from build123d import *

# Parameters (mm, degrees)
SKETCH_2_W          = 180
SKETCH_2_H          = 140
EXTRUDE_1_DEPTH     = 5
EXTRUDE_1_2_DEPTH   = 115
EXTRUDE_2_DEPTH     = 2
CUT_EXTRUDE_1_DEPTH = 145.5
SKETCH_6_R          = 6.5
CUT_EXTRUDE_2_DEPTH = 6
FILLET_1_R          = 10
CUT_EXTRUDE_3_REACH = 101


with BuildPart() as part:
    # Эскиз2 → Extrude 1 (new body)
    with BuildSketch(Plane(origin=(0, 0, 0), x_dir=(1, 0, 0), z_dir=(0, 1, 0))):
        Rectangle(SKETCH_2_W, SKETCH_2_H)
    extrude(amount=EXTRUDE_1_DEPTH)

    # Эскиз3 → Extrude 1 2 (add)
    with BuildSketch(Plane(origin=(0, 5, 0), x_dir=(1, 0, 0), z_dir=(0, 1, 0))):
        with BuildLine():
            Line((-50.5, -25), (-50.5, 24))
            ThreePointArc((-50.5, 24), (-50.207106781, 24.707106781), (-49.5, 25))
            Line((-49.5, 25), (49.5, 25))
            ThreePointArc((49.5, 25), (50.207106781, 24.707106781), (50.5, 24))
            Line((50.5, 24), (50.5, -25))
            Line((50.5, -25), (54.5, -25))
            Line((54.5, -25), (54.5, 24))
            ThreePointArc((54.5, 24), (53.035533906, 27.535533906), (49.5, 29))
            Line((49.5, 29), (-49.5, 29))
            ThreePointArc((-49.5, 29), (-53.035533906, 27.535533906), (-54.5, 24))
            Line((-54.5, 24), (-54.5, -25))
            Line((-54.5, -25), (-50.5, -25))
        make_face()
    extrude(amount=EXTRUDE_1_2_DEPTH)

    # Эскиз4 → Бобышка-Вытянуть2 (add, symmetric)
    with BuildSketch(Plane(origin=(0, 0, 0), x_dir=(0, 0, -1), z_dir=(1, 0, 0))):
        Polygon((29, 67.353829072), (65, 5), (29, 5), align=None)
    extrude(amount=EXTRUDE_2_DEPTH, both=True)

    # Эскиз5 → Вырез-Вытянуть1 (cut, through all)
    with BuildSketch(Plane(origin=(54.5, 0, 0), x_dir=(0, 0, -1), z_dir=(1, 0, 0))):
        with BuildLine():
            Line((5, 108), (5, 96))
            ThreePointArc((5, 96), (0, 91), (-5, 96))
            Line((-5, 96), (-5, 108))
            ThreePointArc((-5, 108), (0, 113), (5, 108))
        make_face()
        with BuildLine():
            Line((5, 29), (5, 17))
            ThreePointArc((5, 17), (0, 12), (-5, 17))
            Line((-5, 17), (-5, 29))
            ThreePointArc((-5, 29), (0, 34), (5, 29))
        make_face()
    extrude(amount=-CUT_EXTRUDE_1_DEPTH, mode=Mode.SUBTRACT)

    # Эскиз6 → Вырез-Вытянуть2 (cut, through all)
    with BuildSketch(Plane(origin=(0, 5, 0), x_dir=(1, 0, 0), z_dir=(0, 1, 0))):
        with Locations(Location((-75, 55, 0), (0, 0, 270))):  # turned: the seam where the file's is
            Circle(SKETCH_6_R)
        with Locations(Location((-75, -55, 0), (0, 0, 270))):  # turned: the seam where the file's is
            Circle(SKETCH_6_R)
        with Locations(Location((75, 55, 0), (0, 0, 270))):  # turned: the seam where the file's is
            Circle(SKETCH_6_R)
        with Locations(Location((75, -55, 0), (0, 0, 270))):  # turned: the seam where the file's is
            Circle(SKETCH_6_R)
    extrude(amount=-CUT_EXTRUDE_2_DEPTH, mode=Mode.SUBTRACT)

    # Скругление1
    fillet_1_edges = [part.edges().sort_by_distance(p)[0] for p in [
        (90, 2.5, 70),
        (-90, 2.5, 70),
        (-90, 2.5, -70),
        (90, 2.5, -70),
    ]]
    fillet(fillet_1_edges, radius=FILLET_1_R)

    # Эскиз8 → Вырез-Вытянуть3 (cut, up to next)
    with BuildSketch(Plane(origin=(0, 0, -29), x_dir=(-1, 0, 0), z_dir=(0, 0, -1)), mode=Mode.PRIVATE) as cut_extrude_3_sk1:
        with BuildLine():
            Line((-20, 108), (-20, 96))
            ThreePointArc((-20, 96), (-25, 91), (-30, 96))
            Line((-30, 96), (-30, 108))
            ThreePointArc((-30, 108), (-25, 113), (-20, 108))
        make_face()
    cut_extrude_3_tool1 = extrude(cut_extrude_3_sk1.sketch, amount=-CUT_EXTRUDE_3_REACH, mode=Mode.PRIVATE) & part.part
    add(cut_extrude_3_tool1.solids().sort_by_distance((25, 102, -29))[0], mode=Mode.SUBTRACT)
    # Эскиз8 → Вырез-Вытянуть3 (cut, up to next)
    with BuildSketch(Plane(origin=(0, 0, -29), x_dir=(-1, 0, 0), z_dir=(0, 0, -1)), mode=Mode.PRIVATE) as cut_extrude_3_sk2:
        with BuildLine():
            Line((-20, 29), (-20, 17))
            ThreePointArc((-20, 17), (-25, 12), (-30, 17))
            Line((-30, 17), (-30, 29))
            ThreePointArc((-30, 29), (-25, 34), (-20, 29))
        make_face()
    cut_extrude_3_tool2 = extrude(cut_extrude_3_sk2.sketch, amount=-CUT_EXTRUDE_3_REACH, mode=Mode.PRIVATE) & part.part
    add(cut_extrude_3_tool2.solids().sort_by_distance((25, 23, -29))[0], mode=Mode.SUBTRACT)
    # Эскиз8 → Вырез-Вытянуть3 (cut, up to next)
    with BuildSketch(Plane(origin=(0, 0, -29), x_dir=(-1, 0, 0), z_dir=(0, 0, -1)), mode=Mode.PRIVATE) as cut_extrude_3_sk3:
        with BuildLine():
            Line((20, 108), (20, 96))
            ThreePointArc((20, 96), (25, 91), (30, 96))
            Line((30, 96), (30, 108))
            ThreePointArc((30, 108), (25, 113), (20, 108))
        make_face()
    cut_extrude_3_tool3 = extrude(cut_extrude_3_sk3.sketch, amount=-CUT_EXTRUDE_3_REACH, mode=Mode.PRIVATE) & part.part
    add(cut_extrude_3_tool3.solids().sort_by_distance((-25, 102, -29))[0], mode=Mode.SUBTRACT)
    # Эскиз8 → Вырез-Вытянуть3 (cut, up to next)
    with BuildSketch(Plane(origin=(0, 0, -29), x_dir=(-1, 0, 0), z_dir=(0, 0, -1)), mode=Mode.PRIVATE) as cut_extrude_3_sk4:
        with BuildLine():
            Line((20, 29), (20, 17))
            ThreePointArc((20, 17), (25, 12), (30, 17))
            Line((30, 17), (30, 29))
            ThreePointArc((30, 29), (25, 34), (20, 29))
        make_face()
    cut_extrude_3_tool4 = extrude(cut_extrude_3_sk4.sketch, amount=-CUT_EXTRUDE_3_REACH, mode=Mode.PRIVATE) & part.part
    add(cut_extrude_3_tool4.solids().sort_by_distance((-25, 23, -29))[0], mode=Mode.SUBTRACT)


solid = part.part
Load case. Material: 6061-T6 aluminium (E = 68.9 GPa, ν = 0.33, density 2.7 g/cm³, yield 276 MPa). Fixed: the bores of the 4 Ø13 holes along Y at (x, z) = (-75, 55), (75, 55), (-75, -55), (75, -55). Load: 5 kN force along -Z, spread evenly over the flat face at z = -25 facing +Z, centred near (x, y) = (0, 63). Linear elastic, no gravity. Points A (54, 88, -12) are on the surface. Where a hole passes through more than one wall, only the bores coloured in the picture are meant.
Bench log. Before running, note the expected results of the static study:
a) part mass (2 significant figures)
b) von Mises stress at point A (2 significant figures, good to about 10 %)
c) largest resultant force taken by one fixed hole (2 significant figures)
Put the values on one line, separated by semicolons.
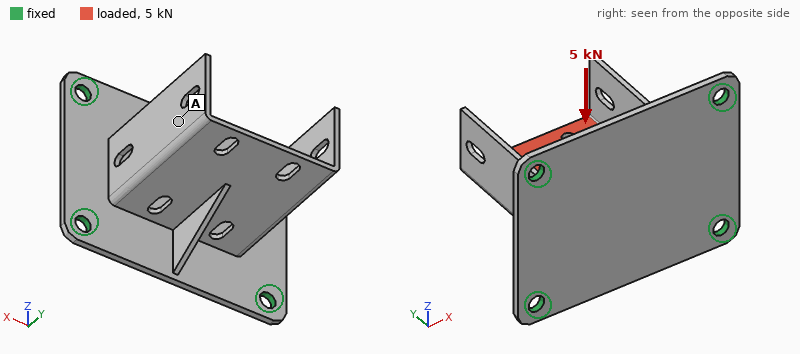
580 g; 50 MPa; 2.2 kN
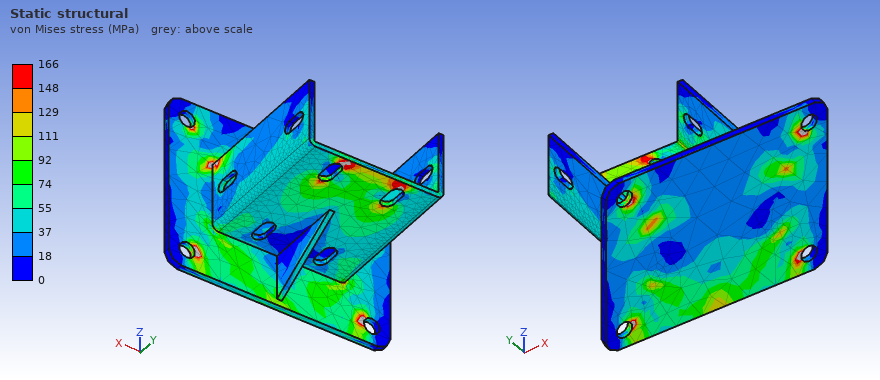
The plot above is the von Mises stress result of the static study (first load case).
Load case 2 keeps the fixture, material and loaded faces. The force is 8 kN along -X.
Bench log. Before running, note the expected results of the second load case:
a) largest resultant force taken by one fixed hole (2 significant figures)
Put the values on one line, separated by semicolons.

4.2 kN
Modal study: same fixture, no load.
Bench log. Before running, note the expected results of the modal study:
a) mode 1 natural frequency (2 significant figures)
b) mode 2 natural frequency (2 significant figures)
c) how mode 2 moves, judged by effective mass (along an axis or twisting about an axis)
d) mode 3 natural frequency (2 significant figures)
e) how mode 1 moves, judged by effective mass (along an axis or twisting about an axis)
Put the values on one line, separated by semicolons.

750 Hz; 790 Hz; along X; 950 Hz; along Z
